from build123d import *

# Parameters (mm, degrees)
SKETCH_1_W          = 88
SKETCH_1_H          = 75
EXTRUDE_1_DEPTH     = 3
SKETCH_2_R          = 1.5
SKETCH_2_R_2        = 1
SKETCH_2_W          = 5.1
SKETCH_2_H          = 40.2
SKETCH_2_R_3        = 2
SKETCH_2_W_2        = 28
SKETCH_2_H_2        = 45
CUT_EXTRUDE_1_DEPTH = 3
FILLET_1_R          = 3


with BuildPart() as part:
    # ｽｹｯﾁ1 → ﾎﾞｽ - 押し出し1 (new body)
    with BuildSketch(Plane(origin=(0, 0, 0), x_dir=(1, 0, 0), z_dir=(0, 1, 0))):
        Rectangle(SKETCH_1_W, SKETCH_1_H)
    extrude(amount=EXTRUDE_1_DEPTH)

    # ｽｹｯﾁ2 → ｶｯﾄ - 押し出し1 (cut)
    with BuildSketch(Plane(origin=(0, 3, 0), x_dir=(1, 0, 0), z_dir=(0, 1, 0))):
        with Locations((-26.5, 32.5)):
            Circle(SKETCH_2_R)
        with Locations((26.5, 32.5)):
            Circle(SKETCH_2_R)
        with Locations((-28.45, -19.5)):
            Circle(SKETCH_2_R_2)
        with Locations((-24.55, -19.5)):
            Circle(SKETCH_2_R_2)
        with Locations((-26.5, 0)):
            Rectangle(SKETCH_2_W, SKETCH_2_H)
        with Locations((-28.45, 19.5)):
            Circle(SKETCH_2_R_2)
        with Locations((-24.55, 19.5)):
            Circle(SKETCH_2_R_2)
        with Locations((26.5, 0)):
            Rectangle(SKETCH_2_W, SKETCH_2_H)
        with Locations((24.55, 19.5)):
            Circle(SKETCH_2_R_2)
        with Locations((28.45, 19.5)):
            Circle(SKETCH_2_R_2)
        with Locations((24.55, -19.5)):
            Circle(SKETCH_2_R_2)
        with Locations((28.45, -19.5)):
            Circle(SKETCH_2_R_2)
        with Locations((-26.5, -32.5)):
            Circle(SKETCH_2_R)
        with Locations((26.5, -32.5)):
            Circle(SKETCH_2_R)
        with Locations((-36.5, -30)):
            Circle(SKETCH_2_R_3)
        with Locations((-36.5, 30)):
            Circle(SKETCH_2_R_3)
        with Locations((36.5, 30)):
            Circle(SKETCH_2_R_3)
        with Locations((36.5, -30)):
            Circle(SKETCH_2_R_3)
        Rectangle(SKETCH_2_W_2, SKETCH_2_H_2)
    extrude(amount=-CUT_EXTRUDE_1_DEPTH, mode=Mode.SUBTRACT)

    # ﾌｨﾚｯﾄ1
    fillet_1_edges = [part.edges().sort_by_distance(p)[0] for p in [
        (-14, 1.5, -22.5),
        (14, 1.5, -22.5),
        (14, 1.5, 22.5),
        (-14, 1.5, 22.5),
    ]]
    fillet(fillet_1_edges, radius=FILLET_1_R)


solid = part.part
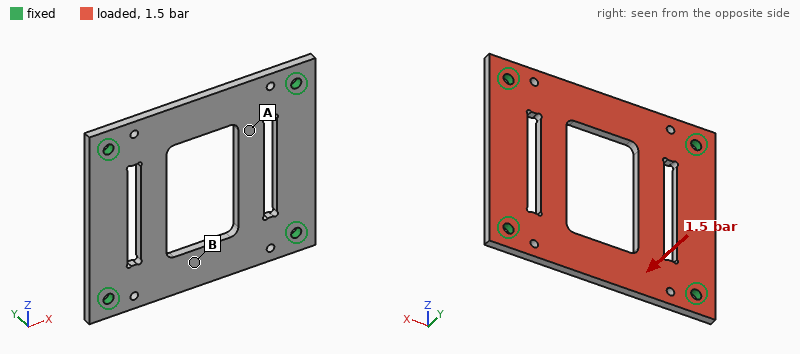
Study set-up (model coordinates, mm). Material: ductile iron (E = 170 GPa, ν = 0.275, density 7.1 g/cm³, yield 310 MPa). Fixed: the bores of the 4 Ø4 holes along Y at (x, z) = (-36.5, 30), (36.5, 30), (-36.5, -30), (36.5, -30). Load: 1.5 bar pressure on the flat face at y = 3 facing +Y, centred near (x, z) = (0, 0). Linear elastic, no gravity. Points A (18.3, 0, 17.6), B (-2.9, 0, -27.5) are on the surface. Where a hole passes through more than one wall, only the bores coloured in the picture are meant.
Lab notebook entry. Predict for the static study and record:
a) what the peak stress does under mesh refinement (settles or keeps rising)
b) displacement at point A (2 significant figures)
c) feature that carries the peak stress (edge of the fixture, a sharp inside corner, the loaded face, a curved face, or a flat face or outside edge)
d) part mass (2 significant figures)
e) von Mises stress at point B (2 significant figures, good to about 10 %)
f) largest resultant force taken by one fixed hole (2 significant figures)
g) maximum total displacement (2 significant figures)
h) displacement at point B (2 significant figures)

keeps rising
29 µm
edge of the fixture
100 g
25 MPa
180 N
45 µm
36 µm
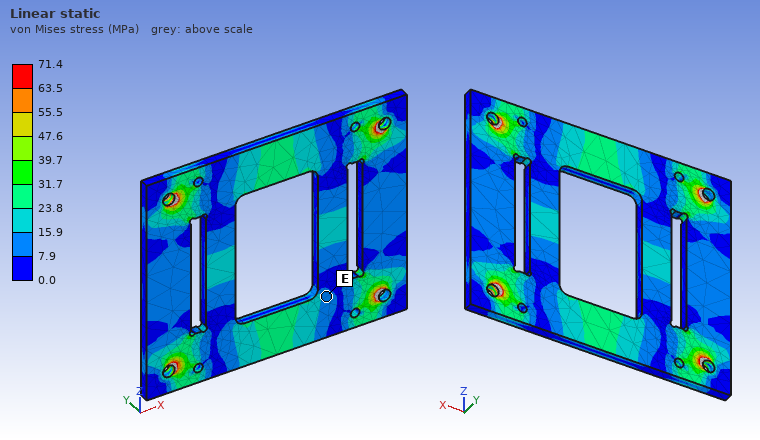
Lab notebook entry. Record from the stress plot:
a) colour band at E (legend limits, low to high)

7.9 to 15.9 MPa
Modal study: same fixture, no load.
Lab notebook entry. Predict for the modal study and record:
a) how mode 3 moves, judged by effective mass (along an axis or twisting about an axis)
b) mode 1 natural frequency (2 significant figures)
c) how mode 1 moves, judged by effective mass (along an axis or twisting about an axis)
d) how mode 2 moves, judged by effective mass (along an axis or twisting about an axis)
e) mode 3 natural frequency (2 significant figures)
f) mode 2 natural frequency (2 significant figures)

twisting about Z
2500 Hz
along Y
twisting about X
3800 Hz
3200 Hz
